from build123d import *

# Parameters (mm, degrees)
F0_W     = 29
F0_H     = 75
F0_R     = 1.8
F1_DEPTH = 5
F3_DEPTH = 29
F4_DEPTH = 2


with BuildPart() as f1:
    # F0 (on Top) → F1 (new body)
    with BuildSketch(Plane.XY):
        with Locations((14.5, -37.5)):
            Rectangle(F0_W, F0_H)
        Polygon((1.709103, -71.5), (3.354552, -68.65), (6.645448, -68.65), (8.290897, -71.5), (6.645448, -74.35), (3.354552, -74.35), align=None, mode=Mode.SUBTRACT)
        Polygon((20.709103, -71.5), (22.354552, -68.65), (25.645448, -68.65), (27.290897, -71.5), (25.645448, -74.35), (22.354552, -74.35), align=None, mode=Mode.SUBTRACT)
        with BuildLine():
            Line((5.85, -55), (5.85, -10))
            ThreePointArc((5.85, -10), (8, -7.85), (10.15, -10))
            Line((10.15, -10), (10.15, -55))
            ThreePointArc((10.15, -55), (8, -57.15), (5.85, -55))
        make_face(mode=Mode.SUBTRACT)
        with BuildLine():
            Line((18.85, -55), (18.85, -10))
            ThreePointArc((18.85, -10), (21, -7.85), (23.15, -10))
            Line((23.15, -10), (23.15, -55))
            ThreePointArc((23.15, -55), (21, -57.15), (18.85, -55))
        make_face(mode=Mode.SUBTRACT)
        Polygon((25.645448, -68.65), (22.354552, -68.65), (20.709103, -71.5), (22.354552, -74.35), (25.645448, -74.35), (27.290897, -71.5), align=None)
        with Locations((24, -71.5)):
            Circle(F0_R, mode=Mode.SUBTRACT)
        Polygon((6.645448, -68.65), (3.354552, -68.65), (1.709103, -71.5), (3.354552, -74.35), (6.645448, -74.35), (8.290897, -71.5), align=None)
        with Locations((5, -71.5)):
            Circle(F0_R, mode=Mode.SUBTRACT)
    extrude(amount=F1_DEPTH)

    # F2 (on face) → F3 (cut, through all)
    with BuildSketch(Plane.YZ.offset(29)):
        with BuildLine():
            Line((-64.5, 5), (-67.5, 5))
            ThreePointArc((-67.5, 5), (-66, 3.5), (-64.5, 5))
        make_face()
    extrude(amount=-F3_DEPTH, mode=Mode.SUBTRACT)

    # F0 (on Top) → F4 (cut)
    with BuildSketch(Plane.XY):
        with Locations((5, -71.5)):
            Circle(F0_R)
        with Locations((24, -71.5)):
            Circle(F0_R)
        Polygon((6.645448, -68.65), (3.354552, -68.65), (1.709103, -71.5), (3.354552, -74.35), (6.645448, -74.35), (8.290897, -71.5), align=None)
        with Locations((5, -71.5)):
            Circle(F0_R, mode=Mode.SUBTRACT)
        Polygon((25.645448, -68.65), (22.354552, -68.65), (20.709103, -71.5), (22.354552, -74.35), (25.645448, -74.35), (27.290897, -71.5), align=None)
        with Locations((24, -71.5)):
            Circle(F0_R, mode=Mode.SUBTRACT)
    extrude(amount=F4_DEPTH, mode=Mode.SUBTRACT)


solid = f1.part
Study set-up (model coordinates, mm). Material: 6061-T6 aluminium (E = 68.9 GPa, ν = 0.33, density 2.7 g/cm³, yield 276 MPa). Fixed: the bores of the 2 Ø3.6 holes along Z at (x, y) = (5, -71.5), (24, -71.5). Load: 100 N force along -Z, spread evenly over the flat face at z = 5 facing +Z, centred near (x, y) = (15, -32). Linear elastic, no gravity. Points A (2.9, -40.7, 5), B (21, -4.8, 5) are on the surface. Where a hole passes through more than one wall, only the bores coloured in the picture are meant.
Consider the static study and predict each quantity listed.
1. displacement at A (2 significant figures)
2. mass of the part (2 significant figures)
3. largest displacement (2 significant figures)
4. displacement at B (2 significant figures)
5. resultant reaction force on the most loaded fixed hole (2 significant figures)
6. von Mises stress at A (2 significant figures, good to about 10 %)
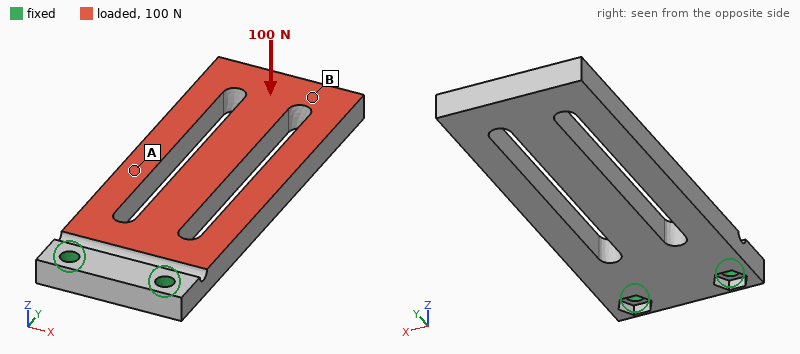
0.14 mm
23 g
0.44 mm
0.41 mm
53 N
16 MPa
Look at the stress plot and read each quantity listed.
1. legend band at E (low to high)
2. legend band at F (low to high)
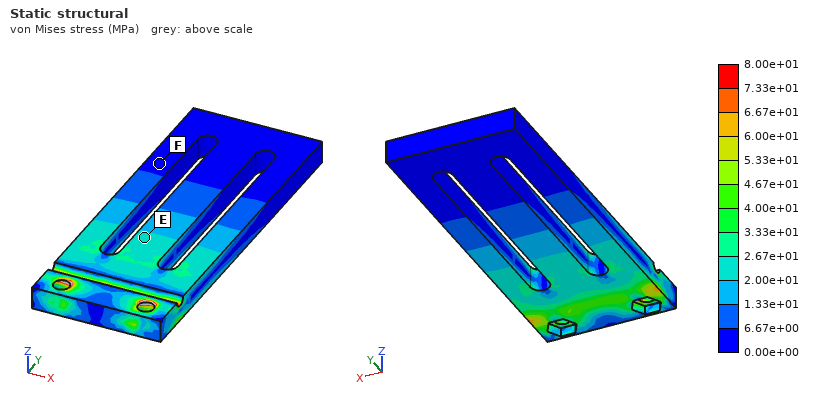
2.00e+01 to 2.67e+01 MPa
0.00e+00 to 6.67e+00 MPa
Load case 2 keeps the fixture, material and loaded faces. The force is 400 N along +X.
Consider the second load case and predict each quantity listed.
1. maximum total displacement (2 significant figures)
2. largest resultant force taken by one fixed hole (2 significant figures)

0.14 mm
770 N
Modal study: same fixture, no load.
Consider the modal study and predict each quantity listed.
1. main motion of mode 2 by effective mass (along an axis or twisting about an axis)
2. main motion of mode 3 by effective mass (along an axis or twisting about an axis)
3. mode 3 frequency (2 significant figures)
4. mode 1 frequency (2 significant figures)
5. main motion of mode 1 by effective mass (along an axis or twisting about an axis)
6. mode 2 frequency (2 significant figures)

along X
twisting about Y
2900 Hz
660 Hz
along Z
2300 Hz
